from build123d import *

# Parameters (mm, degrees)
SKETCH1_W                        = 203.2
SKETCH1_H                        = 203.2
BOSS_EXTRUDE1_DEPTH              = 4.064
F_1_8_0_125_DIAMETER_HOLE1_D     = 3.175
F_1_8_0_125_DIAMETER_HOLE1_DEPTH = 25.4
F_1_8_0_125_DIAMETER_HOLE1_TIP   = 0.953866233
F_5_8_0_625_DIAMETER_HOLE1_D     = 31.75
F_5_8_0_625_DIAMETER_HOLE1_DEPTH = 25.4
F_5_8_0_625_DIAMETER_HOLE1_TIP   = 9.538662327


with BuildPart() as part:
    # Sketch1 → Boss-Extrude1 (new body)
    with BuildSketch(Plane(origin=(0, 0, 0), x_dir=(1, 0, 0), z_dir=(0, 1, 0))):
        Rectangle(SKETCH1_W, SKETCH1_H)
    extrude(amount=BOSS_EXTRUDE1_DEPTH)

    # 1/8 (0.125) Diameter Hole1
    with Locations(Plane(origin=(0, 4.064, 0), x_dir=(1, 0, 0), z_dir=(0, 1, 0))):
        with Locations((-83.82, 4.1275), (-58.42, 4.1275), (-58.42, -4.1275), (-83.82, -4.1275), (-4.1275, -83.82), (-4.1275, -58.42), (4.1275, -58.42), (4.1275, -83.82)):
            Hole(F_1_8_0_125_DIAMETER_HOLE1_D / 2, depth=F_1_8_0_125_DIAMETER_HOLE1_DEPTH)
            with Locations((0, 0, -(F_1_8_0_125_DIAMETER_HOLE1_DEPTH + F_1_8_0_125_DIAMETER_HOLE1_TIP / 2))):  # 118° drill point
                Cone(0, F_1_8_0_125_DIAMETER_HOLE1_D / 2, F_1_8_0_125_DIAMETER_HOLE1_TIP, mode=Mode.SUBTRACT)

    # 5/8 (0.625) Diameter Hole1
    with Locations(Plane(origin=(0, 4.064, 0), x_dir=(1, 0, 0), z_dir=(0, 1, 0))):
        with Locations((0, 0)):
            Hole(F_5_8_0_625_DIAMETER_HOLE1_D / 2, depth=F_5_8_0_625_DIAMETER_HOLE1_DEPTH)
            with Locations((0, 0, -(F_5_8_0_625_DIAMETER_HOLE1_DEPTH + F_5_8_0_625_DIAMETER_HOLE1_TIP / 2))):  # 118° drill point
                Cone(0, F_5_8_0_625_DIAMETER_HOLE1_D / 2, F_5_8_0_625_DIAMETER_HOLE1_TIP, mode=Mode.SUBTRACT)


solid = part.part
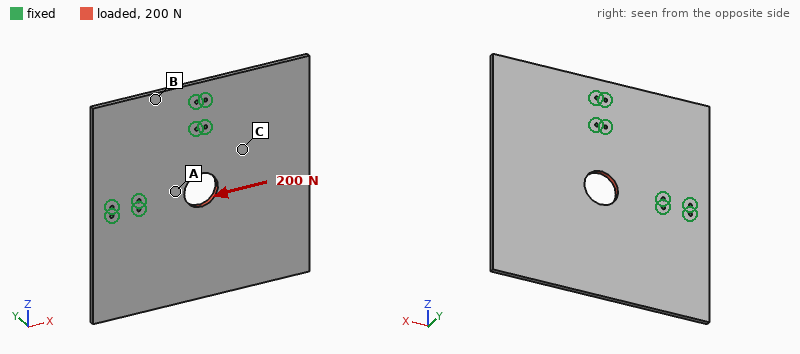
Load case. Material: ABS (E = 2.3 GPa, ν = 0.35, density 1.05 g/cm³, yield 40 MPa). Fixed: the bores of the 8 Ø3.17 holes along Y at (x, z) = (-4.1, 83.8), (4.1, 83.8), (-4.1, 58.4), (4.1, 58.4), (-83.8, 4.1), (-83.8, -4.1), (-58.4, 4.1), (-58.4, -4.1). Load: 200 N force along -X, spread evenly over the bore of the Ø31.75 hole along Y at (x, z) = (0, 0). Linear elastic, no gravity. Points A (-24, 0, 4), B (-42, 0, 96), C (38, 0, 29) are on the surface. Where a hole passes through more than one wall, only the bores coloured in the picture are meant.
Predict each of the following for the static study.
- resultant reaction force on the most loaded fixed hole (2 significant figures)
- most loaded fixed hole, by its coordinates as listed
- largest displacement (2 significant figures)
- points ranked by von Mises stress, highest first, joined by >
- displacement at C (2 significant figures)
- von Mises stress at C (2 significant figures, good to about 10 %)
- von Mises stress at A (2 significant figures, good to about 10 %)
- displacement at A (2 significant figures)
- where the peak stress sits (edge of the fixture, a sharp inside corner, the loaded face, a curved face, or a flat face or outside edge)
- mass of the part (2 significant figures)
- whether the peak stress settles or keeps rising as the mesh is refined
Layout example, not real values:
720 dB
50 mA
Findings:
63 N
(-58.4, -4.1)
32 µm
A > C > B
17 µm
0.24 MPa
0.64 MPa
11 µm
edge of the fixture
170 g
keeps rising
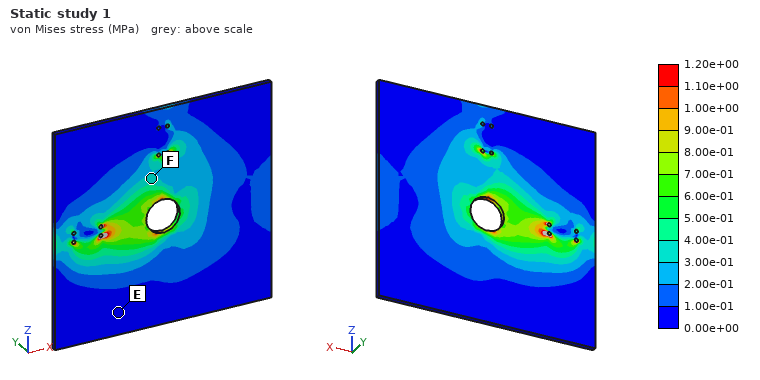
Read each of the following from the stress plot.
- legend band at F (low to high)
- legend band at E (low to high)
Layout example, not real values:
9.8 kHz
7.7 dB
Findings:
3.00e-01 to 4.00e-01 MPa
0.00e+00 to 1.00e-01 MPa
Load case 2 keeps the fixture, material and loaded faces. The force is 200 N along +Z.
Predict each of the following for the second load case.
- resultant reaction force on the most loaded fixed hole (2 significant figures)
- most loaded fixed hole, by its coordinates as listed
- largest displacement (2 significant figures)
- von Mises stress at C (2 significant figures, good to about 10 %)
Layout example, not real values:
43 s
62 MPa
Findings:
63 N
(4.1, 58.4)
32 µm
0.26 MPa
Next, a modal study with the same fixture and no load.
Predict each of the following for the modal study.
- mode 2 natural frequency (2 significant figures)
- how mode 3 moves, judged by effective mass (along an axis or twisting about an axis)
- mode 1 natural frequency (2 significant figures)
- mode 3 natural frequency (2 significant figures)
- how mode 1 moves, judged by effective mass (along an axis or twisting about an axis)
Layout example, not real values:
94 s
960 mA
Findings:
95 Hz
along Y
45 Hz
140 Hz
along Y
